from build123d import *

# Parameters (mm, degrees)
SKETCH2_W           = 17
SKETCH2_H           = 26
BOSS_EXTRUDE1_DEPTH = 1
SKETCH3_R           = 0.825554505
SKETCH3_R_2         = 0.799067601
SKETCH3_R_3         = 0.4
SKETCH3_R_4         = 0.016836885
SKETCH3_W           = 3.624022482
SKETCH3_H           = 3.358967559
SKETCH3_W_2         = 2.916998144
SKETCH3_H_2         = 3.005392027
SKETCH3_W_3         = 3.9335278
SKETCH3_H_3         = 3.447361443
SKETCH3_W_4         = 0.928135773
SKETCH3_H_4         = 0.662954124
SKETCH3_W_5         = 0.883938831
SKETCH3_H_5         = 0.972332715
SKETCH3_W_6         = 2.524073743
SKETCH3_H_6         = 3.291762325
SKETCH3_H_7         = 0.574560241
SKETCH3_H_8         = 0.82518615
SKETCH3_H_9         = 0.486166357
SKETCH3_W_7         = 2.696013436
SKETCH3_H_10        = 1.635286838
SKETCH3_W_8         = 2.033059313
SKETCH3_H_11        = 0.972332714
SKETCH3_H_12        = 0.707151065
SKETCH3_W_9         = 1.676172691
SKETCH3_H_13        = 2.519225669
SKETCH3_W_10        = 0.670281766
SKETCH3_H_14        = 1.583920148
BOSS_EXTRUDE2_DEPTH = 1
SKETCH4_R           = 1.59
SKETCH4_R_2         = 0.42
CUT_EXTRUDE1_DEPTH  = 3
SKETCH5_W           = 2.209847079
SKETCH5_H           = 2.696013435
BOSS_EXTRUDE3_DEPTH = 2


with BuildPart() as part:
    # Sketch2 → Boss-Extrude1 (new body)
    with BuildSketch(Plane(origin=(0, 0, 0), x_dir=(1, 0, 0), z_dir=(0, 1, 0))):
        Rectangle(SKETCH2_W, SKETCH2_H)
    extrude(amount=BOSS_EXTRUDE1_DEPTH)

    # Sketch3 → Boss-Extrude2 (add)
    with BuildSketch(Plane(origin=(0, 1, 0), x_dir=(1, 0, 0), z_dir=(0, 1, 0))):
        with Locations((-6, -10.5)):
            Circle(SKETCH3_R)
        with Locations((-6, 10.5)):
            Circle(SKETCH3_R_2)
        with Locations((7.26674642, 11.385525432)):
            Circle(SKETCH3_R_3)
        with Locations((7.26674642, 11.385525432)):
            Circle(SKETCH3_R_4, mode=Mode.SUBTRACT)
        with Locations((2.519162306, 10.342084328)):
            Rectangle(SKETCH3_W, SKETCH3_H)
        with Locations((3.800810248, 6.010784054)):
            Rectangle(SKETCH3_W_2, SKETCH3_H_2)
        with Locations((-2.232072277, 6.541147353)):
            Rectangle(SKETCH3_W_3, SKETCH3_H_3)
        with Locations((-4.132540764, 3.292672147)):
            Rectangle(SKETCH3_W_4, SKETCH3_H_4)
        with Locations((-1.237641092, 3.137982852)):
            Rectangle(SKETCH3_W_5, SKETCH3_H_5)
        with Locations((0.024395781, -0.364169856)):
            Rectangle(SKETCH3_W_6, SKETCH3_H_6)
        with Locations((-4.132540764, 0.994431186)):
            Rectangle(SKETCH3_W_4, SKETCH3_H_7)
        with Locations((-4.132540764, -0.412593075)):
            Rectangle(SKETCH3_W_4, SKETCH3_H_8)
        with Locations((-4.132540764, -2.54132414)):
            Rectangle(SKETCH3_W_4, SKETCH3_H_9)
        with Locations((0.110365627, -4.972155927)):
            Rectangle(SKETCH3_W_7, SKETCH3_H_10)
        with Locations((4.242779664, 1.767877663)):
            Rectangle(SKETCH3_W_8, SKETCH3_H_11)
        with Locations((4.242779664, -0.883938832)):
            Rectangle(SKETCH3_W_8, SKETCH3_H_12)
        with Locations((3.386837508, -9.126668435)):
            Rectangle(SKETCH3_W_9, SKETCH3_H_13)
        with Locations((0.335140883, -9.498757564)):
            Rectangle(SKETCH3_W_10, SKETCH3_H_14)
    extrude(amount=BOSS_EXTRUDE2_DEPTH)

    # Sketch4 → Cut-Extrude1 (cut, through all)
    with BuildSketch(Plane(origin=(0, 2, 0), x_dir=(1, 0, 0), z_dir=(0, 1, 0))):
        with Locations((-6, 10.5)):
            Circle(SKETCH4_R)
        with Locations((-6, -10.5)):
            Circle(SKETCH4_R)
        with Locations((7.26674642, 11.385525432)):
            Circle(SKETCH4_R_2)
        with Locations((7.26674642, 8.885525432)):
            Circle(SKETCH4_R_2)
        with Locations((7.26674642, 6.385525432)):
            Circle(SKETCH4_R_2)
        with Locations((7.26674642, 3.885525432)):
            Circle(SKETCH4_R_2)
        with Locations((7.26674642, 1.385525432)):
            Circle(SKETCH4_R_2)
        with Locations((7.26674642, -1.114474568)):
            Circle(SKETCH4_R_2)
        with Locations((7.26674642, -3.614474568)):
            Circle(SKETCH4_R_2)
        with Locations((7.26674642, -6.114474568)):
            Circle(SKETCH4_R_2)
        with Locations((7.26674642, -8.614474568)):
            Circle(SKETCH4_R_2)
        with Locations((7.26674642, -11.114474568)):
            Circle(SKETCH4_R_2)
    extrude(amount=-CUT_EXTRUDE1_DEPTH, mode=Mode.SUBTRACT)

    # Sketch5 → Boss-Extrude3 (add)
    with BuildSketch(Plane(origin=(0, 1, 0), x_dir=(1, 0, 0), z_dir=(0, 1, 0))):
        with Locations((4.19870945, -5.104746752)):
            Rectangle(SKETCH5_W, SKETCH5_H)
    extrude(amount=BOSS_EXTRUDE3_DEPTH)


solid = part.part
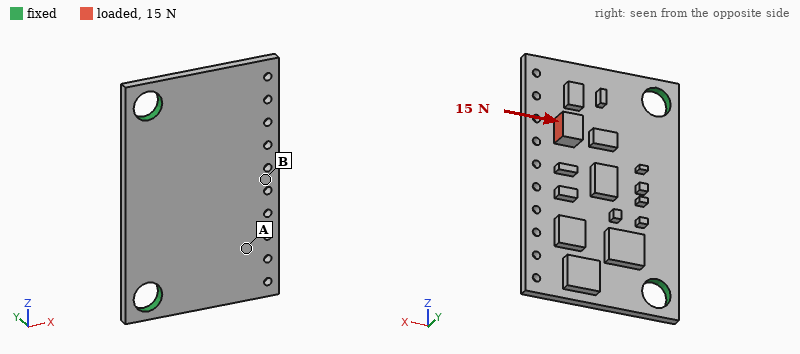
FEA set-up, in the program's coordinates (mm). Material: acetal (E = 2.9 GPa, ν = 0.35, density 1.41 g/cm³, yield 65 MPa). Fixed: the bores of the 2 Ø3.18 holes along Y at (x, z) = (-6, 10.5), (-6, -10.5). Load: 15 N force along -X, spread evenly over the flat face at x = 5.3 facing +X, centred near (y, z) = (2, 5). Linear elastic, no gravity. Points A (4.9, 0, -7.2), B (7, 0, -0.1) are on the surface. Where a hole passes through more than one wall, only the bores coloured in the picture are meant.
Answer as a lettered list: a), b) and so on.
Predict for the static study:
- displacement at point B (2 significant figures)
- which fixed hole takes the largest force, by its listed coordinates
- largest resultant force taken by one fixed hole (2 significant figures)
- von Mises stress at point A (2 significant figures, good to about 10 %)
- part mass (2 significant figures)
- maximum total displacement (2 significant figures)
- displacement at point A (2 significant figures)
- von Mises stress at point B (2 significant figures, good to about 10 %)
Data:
a) 0.26 mm
b) (-6, 10.5)
c) 11 N
d) 1.4 MPa
e) 0.69 g
f) 0.37 mm
g) 0.14 mm
h) 3.7 MPa
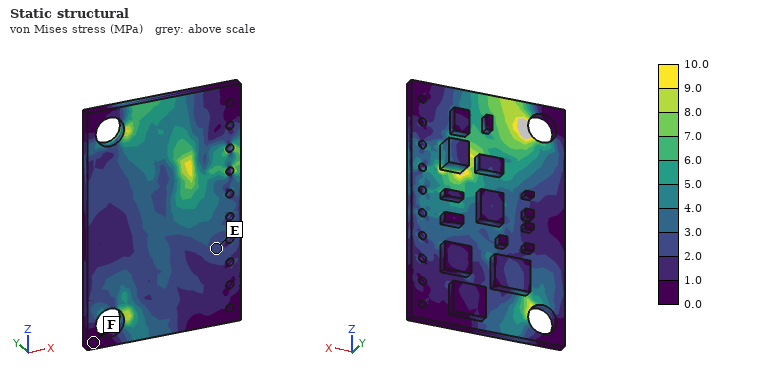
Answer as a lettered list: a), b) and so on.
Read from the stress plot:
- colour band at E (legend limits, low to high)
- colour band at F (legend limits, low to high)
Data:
a) 2.0 to 3.0 MPa
b) 0.0 to 1.0 MPa
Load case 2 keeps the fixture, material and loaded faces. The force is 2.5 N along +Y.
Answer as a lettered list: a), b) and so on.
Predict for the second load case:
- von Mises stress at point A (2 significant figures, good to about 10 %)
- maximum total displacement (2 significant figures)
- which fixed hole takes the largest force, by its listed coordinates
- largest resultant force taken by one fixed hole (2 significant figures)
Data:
a) 1.0 MPa
b) 0.32 mm
c) (-6, 10.5)
d) 2.0 N
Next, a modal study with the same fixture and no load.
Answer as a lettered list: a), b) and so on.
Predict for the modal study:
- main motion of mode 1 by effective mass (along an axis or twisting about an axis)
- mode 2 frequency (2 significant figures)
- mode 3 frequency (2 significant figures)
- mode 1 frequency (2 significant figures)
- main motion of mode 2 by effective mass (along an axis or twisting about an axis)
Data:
a) along Y
b) 2200 Hz
c) 3500 Hz
d) 1100 Hz
e) twisting about X
